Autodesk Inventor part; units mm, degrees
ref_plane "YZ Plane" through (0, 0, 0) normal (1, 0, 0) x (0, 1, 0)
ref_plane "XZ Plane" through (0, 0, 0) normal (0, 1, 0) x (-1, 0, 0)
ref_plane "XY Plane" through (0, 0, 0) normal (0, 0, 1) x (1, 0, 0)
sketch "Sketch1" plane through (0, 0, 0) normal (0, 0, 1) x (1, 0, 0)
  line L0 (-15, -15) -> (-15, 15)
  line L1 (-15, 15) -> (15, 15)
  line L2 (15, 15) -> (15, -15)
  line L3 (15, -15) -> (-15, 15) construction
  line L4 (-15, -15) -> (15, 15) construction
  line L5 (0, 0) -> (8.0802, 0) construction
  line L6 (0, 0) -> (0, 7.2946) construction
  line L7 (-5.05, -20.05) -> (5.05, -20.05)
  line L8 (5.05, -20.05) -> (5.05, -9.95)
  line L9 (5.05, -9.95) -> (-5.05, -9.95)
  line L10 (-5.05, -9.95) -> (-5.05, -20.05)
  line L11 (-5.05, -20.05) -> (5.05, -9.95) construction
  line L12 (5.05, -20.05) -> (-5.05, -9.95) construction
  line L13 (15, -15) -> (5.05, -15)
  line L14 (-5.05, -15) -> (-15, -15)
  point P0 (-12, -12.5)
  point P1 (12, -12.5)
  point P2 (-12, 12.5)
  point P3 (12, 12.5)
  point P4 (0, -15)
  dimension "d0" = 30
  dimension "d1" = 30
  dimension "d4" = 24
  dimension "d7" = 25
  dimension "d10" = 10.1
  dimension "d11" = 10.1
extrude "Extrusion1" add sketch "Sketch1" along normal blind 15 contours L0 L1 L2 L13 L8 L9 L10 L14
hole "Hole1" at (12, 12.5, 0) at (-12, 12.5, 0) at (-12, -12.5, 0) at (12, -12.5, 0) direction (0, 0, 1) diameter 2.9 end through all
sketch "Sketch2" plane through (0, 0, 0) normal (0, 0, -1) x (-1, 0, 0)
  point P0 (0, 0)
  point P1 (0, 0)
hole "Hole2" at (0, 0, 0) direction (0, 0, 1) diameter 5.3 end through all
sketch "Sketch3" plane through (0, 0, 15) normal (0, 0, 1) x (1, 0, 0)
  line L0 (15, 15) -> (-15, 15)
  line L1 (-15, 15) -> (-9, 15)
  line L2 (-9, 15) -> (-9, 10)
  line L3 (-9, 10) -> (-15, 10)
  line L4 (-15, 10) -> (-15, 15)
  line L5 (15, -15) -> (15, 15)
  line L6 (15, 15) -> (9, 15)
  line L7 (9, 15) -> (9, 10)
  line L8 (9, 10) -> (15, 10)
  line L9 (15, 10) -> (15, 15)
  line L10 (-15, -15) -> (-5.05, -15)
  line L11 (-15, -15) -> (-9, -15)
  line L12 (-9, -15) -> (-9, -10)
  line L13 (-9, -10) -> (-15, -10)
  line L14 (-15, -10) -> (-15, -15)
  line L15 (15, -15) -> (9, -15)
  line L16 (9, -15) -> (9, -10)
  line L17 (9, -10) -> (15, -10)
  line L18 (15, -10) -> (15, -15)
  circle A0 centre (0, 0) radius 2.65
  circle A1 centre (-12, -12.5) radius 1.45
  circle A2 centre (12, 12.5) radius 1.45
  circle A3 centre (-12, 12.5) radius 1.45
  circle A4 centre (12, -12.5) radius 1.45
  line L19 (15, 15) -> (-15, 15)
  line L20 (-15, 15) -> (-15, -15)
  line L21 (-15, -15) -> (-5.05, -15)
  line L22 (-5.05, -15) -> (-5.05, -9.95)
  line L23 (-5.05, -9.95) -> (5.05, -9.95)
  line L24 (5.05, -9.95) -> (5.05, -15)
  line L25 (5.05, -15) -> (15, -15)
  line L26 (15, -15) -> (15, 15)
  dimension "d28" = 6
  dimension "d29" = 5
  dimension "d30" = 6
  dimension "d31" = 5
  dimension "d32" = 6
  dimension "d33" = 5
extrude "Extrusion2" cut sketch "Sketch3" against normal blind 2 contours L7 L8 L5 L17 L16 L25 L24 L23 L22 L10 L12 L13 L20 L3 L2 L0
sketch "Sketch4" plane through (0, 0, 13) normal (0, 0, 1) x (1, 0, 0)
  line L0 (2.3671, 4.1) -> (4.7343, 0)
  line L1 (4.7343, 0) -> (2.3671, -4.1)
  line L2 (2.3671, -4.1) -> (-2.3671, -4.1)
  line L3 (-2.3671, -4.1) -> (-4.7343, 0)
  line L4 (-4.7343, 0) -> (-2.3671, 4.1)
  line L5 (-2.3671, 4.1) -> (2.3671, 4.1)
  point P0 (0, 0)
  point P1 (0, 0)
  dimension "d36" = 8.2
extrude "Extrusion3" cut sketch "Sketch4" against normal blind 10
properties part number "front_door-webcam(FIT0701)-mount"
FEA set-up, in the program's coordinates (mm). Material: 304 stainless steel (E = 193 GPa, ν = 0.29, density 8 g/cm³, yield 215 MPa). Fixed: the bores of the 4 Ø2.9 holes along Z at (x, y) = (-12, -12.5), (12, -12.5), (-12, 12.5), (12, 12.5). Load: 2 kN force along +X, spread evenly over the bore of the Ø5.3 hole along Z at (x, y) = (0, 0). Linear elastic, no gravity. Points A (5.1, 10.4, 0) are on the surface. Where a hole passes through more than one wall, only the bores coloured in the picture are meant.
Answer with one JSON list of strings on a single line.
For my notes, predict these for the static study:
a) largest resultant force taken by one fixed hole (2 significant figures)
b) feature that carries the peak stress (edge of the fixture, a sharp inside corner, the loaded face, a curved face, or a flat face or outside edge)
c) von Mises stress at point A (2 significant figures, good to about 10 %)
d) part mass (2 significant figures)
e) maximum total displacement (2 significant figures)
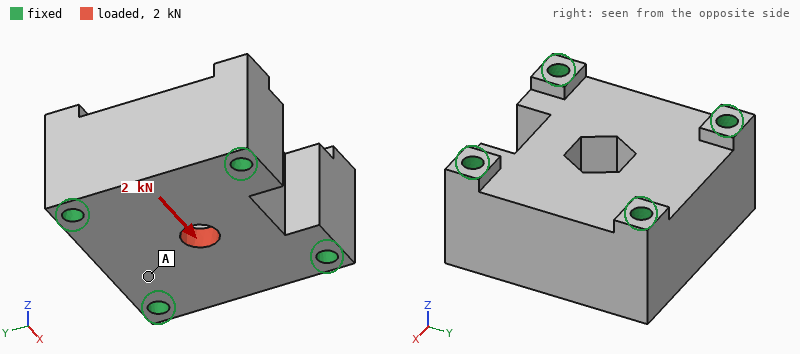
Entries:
["650 N", "a sharp inside corner", "7.0 MPa", "82 g", "1.7 µm"]
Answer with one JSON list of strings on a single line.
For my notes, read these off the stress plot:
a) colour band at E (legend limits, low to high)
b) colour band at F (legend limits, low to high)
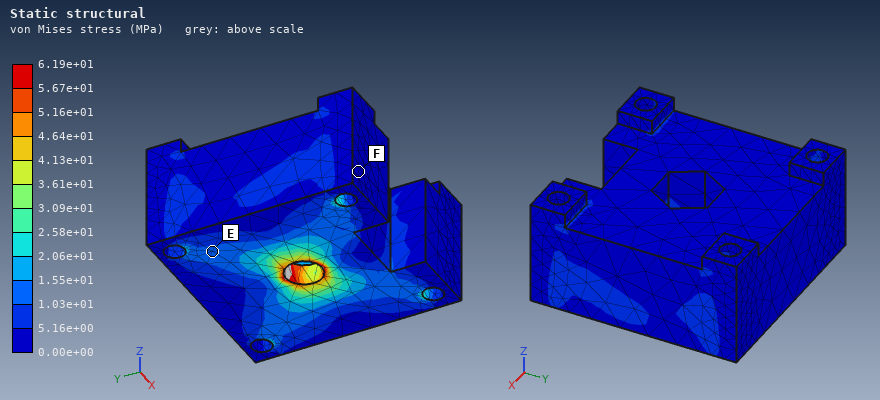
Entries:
["1.03e+01 to 1.55e+01 MPa", "0.00e+00 to 5.16e+00 MPa"]
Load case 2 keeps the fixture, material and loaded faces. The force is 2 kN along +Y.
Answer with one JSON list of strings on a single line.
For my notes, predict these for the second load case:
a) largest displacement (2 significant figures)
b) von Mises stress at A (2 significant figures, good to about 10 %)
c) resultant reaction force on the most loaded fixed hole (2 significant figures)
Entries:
["1.8 µm", "10 MPa", "610 N"]
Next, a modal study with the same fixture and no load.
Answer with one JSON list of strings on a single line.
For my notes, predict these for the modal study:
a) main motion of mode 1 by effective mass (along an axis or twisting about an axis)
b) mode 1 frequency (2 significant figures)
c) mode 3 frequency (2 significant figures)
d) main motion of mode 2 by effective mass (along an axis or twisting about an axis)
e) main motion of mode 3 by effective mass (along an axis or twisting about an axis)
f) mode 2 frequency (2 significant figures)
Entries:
["along Z", "41 kHz", "53 kHz", "along X", "twisting about Y", "49 kHz"]
